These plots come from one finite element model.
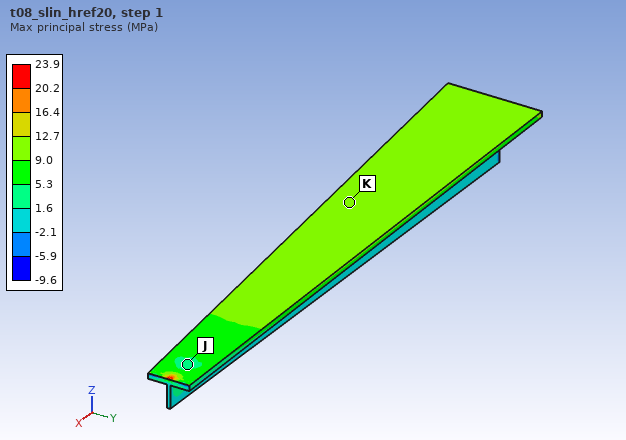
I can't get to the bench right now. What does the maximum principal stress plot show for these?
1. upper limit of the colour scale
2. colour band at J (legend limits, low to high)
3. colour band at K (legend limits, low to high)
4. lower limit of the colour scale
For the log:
23.9 MPa
1.6 to 5.3 MPa
9.0 to 12.7 MPa
-9.6 MPa
